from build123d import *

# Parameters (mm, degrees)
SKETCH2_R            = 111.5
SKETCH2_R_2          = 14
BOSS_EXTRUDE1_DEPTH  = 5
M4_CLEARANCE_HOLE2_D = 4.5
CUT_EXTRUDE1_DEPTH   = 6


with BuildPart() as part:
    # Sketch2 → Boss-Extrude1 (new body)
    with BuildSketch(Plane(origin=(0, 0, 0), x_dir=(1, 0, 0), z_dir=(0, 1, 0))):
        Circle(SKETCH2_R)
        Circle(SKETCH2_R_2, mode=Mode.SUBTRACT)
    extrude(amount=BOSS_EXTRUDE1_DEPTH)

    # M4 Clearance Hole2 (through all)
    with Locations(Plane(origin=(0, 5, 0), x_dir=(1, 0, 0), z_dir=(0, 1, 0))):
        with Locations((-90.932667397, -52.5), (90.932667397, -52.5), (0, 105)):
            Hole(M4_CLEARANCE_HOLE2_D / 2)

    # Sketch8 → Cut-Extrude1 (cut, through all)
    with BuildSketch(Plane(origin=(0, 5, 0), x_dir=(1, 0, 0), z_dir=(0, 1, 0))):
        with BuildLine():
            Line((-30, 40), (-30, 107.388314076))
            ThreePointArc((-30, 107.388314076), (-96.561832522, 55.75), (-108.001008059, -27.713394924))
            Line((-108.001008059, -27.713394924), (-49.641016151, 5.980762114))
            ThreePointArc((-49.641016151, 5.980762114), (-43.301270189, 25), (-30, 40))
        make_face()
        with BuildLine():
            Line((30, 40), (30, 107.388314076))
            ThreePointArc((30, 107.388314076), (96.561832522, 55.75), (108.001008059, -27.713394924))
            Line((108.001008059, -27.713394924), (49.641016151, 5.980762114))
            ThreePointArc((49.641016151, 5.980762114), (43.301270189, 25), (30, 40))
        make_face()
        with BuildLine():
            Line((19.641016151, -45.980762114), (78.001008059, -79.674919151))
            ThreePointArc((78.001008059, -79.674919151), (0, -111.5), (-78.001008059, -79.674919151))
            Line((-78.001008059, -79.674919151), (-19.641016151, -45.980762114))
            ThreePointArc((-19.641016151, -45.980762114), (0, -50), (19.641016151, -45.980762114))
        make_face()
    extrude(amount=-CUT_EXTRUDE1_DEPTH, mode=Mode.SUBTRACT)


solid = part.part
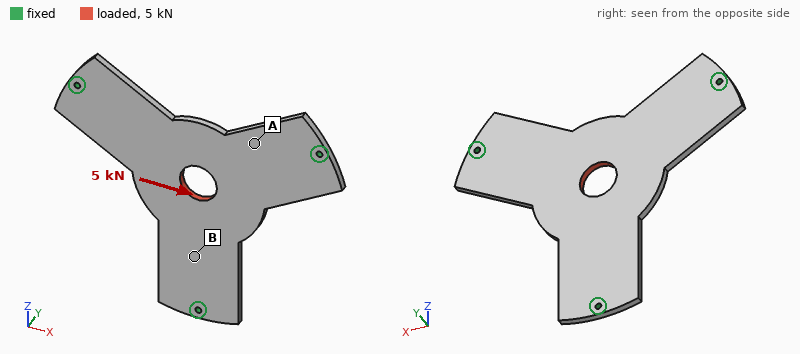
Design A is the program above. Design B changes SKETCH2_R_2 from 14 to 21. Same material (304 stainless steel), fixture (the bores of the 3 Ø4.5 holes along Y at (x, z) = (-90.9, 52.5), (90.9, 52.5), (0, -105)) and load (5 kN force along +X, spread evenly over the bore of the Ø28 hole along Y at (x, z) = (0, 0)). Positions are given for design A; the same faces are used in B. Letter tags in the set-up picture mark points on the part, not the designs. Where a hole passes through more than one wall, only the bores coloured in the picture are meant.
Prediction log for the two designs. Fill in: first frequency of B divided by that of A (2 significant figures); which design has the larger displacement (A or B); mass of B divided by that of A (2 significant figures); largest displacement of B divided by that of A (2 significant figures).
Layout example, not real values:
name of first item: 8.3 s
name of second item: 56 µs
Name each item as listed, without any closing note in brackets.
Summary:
first frequency of B divided by that of A: 1.0
which design has the larger displacement: B
mass of B divided by that of A: 0.96
largest displacement of B divided by that of A: 1.2
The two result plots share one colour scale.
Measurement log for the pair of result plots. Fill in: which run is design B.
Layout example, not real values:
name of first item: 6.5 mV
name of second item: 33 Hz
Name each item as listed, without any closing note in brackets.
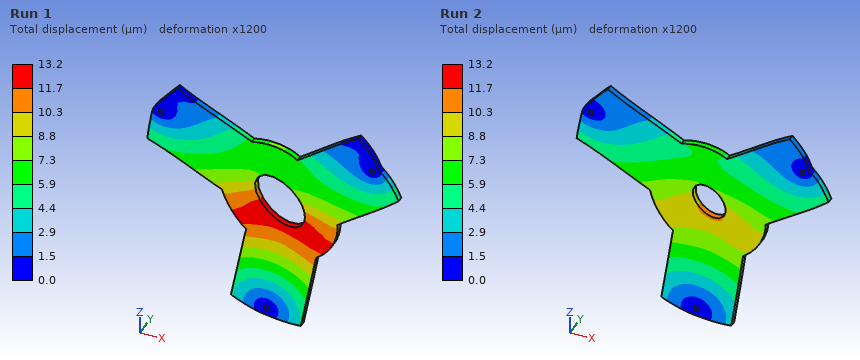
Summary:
which run is design B: Run 1
